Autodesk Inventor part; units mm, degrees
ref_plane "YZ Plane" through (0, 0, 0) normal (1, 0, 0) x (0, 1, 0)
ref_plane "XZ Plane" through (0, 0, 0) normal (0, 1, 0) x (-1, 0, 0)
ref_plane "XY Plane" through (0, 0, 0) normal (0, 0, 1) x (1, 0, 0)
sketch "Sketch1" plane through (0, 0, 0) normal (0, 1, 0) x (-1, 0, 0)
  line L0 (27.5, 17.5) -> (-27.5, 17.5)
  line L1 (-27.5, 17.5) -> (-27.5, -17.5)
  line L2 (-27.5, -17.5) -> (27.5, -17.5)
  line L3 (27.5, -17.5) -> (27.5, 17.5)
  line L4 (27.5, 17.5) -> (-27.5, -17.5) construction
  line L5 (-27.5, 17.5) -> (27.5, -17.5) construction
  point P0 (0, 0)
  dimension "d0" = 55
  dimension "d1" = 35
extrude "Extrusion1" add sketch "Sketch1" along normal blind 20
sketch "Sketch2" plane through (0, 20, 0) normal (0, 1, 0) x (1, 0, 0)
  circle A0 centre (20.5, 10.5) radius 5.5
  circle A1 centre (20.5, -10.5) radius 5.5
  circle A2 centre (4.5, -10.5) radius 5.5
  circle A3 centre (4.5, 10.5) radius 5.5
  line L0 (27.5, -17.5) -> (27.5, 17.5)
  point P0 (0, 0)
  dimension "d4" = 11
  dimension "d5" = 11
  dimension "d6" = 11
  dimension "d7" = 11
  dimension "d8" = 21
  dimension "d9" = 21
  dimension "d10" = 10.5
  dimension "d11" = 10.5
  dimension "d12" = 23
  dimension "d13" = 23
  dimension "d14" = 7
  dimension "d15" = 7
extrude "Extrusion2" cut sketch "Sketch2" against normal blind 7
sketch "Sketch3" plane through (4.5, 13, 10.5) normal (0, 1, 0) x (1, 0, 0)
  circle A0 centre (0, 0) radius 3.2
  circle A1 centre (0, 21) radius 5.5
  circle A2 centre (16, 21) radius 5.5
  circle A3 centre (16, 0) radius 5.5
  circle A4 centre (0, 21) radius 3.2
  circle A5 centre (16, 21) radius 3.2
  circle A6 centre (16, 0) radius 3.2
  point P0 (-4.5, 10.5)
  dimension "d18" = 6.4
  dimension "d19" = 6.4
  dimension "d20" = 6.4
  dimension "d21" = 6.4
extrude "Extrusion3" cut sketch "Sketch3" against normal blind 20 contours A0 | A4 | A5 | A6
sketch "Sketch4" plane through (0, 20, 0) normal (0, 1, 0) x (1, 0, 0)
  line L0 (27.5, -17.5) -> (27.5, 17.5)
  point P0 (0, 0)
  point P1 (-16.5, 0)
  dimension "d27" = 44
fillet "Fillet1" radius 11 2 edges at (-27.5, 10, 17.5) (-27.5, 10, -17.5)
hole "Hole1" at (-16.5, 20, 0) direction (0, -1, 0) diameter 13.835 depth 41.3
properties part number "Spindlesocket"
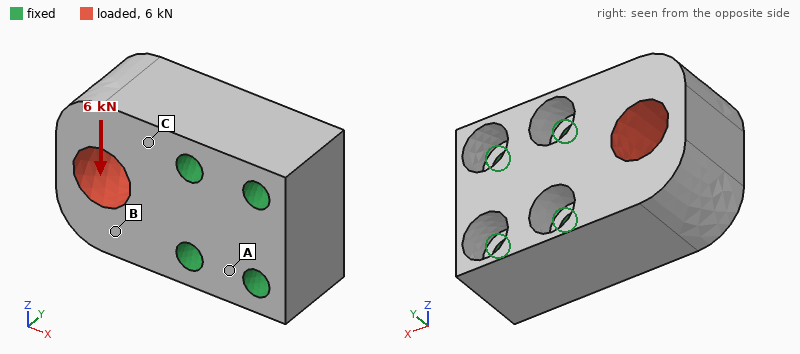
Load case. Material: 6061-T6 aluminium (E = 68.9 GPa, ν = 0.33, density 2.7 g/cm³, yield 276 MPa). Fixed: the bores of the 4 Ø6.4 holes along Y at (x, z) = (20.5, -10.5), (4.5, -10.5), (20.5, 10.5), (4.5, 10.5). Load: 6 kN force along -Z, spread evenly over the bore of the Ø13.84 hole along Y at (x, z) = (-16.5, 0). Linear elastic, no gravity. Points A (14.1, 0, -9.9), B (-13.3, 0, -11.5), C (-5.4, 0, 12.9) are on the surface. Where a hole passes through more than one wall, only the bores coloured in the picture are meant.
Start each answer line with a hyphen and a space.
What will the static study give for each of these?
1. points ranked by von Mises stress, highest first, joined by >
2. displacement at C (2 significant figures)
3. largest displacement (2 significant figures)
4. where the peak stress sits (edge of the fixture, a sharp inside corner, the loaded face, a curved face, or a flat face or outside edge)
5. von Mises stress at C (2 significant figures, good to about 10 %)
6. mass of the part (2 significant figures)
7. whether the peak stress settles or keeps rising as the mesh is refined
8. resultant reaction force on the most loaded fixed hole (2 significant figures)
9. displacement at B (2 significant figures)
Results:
- B > C > A
- 5.9 µm
- 28 µm
- edge of the fixture
- 15 MPa
- 81 g
- keeps rising
- 5.2 kN
- 13 µm
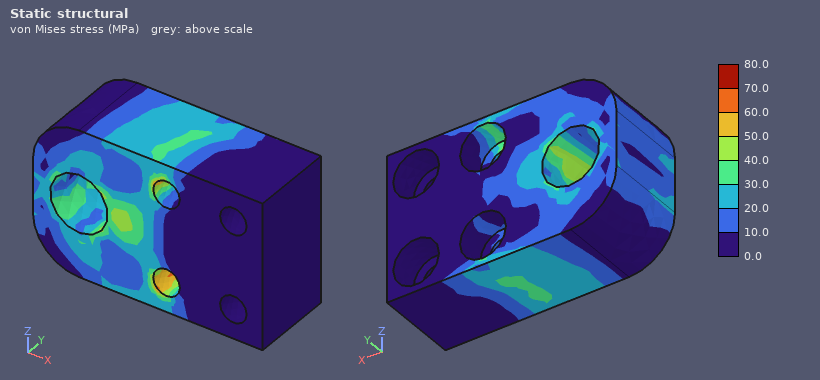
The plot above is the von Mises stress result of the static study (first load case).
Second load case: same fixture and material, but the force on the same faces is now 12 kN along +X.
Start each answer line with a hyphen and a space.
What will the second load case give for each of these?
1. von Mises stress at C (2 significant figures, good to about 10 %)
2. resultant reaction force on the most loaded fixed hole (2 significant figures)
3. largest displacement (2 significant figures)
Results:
- 15 MPa
- 5.1 kN
- 25 µm
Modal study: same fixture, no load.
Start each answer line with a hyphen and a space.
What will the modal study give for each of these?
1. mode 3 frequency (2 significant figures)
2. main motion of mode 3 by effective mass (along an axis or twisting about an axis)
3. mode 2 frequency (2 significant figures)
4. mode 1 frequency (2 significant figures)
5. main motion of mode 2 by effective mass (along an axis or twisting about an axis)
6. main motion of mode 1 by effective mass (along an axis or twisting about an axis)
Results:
- 19 kHz
- twisting about X
- 16 kHz
- 11 kHz
- along Z
- along Y
